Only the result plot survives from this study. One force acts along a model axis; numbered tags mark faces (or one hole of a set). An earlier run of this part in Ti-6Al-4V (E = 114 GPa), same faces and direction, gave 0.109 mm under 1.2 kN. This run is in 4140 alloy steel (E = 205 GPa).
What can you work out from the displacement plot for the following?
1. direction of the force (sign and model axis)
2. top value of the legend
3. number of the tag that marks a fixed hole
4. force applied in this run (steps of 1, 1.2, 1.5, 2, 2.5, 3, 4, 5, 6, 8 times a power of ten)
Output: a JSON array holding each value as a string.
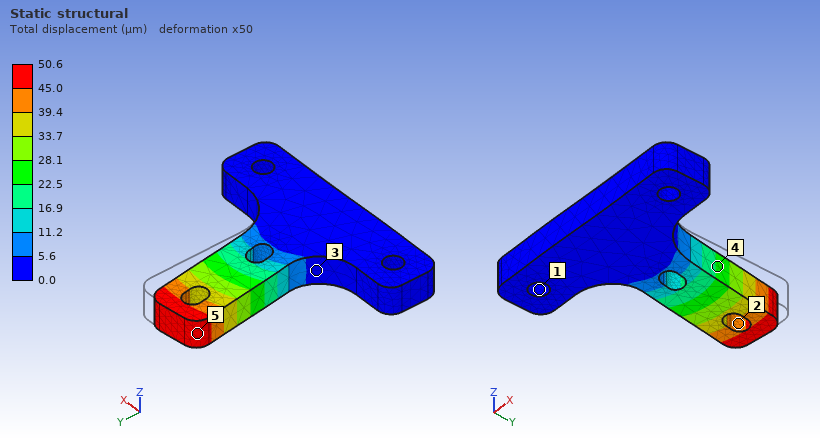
["-X", "50.6 µm", "1", "1 kN"]
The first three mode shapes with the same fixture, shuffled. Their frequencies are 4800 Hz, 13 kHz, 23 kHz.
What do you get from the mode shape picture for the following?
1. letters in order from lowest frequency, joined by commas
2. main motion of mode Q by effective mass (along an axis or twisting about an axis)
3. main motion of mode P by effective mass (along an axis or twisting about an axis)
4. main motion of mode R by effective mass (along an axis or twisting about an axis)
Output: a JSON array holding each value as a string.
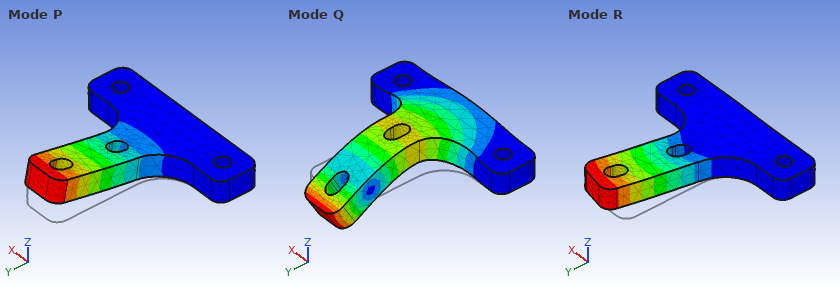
["P, R, Q", "along Z", "along Z", "along X"]
